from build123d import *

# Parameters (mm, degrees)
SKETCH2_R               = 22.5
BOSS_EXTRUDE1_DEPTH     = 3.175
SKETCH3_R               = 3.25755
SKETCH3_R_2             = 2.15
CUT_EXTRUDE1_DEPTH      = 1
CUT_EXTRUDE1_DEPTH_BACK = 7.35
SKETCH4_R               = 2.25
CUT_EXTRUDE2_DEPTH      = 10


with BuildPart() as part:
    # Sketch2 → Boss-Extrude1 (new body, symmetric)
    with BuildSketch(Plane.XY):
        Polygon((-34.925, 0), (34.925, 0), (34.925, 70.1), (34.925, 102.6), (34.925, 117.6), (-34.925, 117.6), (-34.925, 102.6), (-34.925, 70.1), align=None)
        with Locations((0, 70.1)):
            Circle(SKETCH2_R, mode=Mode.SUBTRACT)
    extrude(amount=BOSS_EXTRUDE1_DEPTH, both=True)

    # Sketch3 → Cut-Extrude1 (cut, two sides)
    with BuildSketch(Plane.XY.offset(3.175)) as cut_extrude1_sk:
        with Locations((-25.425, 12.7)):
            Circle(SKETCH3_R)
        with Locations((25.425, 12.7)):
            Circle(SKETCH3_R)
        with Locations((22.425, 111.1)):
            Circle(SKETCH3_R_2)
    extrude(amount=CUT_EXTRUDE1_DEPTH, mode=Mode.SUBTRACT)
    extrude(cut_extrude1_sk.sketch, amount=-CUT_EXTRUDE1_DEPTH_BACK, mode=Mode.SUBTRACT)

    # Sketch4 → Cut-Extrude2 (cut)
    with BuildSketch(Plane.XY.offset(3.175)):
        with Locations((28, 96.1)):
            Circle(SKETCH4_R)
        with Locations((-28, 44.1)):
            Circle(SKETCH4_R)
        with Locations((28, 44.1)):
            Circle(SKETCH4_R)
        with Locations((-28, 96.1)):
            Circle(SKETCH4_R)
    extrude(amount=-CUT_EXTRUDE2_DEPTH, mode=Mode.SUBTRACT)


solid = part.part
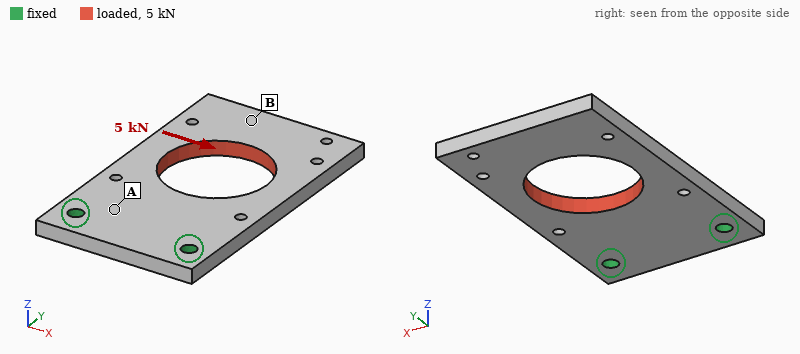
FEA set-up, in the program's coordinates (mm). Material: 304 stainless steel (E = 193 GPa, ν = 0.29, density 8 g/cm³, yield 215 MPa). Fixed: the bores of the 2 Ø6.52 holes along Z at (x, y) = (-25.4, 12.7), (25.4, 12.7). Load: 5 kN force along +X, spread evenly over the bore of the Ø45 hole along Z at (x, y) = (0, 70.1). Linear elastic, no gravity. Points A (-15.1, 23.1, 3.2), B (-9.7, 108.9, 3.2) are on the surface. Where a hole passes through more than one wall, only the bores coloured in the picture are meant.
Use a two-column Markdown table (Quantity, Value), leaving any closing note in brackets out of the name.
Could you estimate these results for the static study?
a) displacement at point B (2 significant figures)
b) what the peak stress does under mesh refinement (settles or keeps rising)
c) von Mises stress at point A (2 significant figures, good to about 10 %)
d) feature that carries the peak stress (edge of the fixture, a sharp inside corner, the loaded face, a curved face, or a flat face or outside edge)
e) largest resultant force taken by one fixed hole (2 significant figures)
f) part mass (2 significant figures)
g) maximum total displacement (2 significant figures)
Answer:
| Quantity | Value |
|---|---|
| displacement at point B | 68 µm |
| what the peak stress does under mesh refinement | keeps rising |
| von Mises stress at point A | 30 MPa |
| feature that carries the peak stress | edge of the fixture |
| largest resultant force taken by one fixed hole | 5.9 kN |
| part mass | 330 g |
| maximum total displacement | 72 µm |
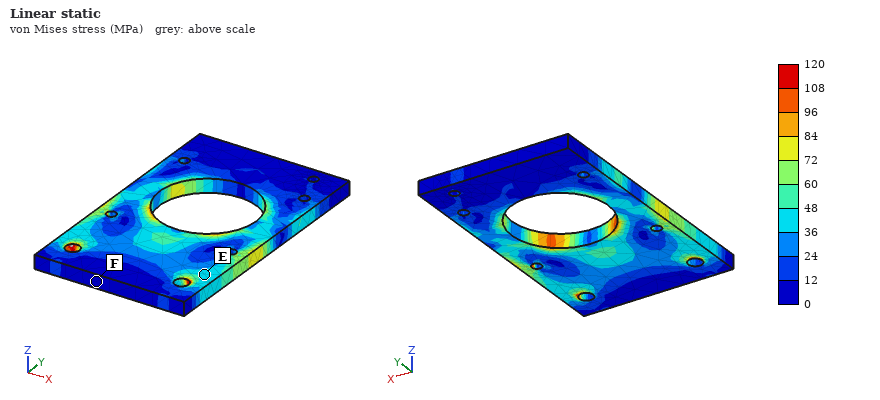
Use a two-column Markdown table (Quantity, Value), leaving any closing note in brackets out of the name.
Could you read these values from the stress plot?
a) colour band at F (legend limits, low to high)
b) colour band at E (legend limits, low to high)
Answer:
| Quantity | Value |
|---|---|
| colour band at F | 0 to 12 MPa |
| colour band at E | 36 to 48 MPa |
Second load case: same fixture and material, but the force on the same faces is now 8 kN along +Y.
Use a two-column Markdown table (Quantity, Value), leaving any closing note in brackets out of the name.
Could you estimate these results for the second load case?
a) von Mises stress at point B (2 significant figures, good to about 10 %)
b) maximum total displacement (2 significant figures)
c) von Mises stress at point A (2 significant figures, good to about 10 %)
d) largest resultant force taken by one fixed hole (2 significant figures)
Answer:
| Quantity | Value |
|---|---|
| von Mises stress at point B | 11 MPa |
| maximum total displacement | 16 µm |
| von Mises stress at point A | 15 MPa |
| largest resultant force taken by one fixed hole | 4.0 kN |
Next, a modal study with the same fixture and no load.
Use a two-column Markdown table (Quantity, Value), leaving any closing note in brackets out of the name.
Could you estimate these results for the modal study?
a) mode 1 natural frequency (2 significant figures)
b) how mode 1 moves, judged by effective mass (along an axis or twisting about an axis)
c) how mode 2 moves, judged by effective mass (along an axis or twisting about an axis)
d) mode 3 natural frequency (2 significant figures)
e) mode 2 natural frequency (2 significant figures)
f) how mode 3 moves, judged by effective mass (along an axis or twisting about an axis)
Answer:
| Quantity | Value |
|---|---|
| mode 1 natural frequency | 420 Hz |
| how mode 1 moves, judged by effective mass | along Z |
| how mode 2 moves, judged by effective mass | twisting about Y |
| mode 3 natural frequency | 2600 Hz |
| mode 2 natural frequency | 1300 Hz |
| how mode 3 moves, judged by effective mass | along Z |
